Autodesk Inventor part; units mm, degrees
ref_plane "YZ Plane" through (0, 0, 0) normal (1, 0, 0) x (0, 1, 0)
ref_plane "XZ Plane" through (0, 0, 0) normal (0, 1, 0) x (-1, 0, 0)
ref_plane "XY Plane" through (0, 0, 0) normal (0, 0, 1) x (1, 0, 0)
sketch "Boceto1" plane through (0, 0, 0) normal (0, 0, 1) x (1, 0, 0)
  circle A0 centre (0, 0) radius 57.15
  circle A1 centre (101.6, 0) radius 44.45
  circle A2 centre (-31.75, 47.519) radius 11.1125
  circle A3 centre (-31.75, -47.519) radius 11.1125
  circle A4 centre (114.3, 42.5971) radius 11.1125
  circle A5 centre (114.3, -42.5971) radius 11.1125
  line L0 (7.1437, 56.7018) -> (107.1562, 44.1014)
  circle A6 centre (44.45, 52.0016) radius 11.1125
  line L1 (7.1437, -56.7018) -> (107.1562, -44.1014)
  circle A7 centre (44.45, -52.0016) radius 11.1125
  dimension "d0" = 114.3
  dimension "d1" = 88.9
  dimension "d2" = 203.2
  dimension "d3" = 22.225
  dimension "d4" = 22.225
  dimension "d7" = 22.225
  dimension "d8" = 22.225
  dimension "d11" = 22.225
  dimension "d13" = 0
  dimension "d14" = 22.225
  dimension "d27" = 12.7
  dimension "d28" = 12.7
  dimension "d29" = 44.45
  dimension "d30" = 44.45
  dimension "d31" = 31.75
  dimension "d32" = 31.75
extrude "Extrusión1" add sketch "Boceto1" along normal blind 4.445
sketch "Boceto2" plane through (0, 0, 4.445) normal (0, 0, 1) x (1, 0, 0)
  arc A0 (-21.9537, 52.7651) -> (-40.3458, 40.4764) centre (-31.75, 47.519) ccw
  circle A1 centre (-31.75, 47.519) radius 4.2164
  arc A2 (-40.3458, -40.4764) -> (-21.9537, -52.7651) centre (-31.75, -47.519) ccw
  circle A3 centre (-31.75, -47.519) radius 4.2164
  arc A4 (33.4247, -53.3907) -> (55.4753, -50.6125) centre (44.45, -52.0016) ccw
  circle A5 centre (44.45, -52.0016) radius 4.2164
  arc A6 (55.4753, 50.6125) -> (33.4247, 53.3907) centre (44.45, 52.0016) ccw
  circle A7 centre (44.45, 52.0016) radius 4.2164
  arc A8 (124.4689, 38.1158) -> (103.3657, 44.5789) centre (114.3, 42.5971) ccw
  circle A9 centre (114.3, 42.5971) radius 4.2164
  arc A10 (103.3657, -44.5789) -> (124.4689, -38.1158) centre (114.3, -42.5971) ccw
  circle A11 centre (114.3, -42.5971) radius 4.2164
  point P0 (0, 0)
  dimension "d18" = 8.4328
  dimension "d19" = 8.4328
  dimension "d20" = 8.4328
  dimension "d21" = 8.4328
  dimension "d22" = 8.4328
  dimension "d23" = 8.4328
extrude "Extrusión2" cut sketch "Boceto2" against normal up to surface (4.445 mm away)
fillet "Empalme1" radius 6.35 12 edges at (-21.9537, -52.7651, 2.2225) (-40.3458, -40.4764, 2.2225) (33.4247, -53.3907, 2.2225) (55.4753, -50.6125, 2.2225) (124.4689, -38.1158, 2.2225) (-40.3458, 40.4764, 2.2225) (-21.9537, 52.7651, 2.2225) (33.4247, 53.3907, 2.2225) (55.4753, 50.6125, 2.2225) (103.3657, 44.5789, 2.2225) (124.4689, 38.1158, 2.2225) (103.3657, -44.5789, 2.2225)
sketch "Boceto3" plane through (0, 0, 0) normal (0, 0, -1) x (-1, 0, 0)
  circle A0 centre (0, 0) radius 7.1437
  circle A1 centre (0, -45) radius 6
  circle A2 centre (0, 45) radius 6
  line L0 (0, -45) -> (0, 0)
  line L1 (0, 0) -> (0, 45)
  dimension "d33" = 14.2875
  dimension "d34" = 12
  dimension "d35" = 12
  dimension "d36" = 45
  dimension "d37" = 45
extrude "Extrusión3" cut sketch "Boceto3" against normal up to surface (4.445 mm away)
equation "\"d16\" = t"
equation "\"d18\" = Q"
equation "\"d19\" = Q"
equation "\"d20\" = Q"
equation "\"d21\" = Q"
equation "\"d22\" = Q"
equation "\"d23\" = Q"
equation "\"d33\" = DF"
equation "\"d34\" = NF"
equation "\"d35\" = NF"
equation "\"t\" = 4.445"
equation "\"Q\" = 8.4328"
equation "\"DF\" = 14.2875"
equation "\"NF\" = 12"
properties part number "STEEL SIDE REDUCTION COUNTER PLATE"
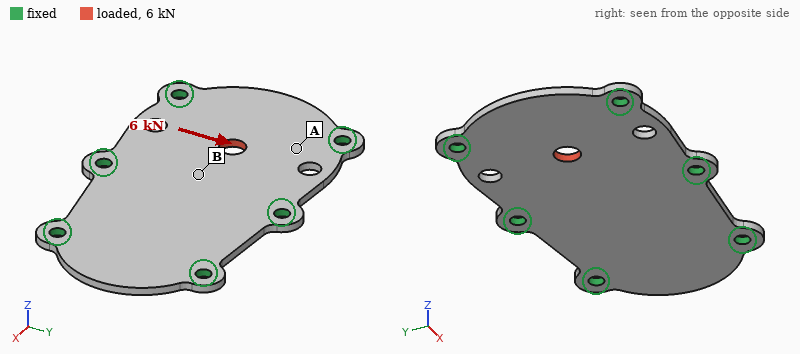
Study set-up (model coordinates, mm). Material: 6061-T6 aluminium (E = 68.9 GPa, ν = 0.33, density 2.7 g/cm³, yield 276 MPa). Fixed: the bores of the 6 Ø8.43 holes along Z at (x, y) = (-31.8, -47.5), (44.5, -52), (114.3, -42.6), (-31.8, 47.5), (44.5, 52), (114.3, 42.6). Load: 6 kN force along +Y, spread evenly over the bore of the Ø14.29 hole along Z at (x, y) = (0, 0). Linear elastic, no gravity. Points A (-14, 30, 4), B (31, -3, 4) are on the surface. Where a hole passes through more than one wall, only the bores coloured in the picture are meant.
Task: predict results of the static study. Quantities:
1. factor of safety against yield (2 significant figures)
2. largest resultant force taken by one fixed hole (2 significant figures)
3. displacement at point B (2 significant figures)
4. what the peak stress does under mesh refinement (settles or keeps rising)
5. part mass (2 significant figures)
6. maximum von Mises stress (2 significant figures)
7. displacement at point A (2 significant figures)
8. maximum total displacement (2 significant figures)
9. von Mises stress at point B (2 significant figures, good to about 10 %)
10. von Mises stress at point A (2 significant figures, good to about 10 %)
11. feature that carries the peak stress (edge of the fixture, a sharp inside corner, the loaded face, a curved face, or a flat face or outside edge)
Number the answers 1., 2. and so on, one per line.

1. 5.3
2. 1.8 kN
3. 5.3 µm
4. settles
5. 230 g
6. 52 MPa
7. 6.8 µm
8. 15 µm
9. 6.1 MPa
10. 15 MPa
11. the loaded face
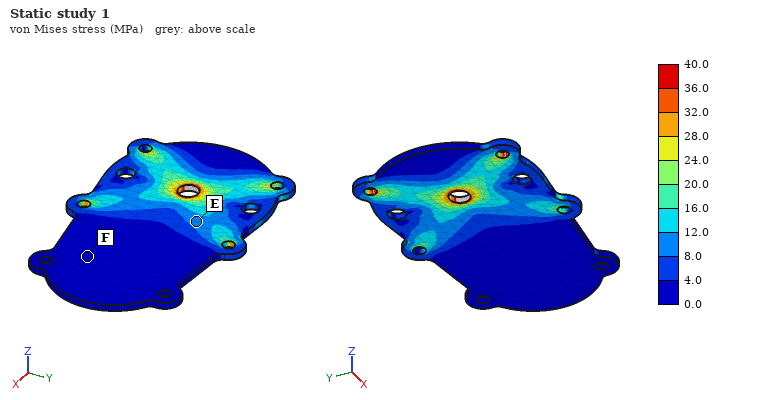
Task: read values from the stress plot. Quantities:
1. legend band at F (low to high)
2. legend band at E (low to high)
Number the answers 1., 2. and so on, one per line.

1. 0.0 to 4.0 MPa
2. 8.0 to 12.0 MPa
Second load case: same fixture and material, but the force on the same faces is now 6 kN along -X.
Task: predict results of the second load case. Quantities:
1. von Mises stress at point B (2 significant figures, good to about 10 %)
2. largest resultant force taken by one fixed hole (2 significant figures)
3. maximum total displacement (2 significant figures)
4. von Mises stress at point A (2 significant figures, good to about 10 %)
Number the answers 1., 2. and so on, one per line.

1. 12 MPa
2. 1.4 kN
3. 18 µm
4. 11 MPa
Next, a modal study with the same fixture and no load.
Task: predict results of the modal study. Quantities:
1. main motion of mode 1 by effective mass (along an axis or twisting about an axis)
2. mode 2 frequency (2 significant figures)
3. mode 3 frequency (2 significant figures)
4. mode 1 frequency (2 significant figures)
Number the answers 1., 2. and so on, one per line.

1. along Z
2. 2500 Hz
3. 2500 Hz
4. 2000 Hz
